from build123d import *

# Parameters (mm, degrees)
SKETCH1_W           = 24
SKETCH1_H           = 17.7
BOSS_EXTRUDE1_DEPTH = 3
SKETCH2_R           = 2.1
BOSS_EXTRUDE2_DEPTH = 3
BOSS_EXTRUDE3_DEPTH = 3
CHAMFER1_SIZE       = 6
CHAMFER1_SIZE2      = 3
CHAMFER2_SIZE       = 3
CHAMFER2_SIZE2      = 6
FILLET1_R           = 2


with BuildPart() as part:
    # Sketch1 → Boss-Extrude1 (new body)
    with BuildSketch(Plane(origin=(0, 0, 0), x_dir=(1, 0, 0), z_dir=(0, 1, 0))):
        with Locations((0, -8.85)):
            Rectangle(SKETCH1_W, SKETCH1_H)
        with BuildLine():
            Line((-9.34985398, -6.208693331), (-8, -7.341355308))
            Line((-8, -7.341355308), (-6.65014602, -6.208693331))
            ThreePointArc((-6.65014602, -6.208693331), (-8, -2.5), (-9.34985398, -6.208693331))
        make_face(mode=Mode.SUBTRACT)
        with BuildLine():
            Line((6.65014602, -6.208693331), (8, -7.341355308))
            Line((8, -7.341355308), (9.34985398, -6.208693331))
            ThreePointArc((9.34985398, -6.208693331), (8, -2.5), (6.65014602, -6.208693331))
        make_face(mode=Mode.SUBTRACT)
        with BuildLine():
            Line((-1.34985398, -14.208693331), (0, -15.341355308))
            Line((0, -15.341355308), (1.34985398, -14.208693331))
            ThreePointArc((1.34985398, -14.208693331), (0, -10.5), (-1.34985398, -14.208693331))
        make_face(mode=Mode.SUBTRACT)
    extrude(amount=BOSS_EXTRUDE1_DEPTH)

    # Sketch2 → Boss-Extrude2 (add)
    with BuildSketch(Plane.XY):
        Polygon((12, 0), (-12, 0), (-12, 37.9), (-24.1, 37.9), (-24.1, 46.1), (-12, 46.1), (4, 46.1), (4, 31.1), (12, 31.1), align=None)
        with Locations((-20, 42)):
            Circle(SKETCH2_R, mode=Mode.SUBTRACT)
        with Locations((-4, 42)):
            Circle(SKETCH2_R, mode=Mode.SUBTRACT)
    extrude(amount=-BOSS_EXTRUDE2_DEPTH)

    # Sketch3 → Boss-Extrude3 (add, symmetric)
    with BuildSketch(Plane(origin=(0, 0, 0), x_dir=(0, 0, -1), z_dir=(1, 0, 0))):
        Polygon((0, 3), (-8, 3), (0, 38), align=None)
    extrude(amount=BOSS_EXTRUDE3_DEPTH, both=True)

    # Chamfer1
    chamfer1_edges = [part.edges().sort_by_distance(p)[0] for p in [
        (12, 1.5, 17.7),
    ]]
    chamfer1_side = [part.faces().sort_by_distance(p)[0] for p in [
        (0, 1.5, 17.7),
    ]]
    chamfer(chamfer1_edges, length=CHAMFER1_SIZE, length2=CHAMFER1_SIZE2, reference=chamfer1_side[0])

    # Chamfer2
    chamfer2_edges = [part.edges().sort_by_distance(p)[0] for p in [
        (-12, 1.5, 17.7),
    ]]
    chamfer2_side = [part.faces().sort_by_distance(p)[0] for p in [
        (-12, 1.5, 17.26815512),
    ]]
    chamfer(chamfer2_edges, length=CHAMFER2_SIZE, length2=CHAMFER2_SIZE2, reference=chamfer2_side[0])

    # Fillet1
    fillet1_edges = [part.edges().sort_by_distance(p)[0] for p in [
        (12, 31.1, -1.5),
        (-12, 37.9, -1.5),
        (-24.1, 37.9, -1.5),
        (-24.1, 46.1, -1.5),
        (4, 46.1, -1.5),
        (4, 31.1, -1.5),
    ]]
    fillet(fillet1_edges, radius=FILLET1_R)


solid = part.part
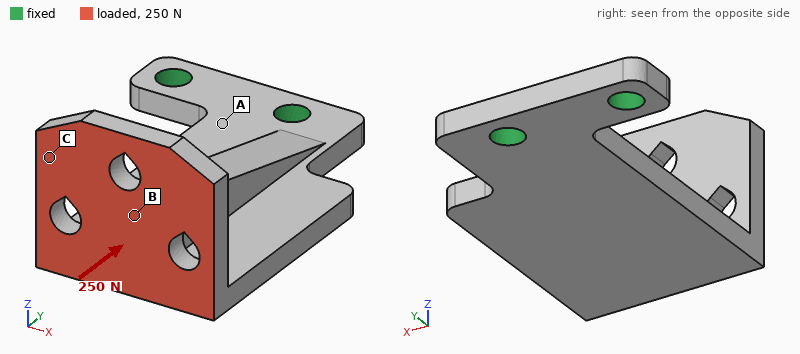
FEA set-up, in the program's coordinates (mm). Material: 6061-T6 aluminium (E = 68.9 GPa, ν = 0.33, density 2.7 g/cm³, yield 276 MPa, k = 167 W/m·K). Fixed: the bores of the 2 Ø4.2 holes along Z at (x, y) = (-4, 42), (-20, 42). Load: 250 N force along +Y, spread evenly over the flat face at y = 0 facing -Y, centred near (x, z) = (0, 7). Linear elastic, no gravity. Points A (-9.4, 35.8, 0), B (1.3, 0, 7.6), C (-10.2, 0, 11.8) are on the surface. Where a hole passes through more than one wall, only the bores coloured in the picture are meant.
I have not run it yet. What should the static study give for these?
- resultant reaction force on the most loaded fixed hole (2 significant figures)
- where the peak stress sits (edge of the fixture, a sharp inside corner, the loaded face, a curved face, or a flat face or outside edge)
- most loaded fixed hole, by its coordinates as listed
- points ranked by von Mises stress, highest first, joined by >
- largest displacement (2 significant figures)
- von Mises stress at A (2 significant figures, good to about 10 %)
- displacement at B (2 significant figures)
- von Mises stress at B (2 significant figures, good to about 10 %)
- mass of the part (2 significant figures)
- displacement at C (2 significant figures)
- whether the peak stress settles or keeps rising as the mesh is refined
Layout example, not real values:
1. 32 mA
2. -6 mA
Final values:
1. 280 N
2. edge of the fixture
3. (-4, 42)
4. A > B > C
5. 0.39 mm
6. 64 MPa
7. 0.34 mm
8. 23 MPa
9. 14 g
10. 0.35 mm
11. keeps rising
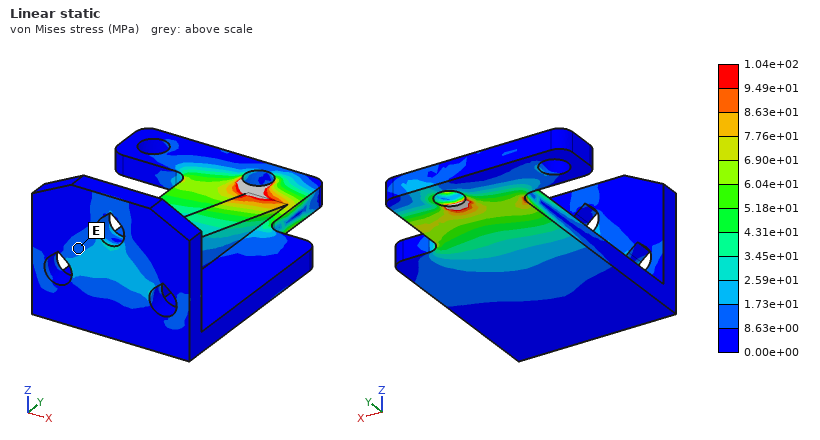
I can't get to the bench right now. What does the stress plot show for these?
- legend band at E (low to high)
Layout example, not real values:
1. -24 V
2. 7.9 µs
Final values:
1. 8.63e+00 to 1.73e+01 MPa
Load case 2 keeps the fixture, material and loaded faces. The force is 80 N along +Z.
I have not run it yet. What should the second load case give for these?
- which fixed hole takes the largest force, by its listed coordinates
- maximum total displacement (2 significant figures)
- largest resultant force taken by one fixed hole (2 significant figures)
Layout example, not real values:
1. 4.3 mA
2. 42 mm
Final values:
1. (-4, 42)
2. 0.52 mm
3. 120 N
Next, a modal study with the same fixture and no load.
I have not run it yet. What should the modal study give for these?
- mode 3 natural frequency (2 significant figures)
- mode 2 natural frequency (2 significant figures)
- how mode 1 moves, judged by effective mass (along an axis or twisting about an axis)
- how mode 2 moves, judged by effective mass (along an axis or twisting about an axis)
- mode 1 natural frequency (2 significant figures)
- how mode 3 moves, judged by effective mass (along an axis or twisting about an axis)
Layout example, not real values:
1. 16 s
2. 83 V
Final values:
1. 3900 Hz
2. 2400 Hz
3. along Z
4. along X
5. 860 Hz
6. along X
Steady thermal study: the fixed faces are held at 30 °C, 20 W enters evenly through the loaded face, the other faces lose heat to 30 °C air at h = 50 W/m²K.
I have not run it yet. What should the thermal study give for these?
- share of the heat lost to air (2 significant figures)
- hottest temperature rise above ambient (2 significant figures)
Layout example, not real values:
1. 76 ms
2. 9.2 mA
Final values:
1. 27 %
2. 59 K
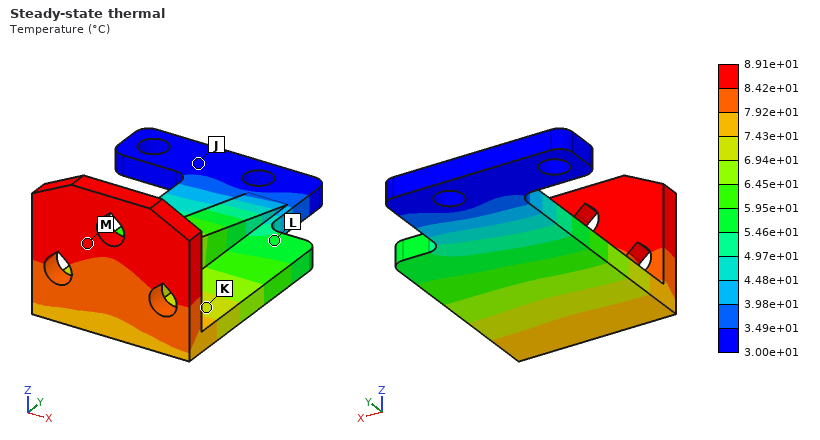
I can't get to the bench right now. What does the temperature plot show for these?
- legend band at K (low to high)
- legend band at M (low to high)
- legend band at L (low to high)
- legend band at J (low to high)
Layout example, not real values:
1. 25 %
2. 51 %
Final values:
1. 6.94e+01 to 7.43e+01 °C
2. 8.42e+01 to 8.91e+01 °C
3. 5.46e+01 to 5.95e+01 °C
4. 3.00e+01 to 3.49e+01 °C
